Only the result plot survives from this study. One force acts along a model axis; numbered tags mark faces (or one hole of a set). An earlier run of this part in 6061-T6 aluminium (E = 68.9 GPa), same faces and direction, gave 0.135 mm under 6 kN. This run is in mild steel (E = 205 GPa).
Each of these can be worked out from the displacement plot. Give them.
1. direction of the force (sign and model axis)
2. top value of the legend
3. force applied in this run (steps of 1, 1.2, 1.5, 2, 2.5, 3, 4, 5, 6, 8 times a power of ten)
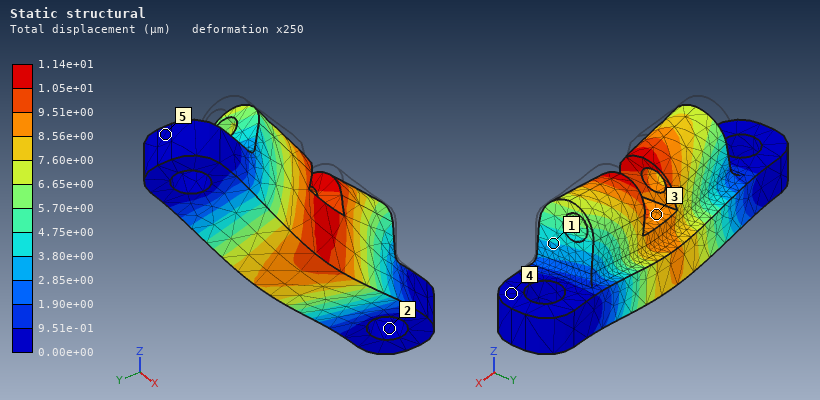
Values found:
-Z
1.14e+01 µm
1.5 kN
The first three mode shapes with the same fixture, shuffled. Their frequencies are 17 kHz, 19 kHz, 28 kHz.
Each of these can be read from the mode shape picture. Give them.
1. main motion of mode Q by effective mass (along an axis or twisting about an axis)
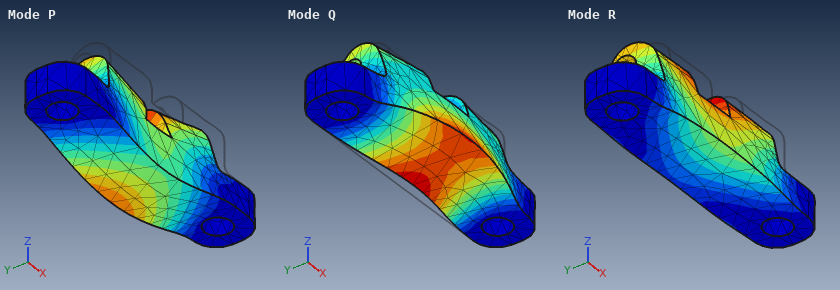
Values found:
along Y
